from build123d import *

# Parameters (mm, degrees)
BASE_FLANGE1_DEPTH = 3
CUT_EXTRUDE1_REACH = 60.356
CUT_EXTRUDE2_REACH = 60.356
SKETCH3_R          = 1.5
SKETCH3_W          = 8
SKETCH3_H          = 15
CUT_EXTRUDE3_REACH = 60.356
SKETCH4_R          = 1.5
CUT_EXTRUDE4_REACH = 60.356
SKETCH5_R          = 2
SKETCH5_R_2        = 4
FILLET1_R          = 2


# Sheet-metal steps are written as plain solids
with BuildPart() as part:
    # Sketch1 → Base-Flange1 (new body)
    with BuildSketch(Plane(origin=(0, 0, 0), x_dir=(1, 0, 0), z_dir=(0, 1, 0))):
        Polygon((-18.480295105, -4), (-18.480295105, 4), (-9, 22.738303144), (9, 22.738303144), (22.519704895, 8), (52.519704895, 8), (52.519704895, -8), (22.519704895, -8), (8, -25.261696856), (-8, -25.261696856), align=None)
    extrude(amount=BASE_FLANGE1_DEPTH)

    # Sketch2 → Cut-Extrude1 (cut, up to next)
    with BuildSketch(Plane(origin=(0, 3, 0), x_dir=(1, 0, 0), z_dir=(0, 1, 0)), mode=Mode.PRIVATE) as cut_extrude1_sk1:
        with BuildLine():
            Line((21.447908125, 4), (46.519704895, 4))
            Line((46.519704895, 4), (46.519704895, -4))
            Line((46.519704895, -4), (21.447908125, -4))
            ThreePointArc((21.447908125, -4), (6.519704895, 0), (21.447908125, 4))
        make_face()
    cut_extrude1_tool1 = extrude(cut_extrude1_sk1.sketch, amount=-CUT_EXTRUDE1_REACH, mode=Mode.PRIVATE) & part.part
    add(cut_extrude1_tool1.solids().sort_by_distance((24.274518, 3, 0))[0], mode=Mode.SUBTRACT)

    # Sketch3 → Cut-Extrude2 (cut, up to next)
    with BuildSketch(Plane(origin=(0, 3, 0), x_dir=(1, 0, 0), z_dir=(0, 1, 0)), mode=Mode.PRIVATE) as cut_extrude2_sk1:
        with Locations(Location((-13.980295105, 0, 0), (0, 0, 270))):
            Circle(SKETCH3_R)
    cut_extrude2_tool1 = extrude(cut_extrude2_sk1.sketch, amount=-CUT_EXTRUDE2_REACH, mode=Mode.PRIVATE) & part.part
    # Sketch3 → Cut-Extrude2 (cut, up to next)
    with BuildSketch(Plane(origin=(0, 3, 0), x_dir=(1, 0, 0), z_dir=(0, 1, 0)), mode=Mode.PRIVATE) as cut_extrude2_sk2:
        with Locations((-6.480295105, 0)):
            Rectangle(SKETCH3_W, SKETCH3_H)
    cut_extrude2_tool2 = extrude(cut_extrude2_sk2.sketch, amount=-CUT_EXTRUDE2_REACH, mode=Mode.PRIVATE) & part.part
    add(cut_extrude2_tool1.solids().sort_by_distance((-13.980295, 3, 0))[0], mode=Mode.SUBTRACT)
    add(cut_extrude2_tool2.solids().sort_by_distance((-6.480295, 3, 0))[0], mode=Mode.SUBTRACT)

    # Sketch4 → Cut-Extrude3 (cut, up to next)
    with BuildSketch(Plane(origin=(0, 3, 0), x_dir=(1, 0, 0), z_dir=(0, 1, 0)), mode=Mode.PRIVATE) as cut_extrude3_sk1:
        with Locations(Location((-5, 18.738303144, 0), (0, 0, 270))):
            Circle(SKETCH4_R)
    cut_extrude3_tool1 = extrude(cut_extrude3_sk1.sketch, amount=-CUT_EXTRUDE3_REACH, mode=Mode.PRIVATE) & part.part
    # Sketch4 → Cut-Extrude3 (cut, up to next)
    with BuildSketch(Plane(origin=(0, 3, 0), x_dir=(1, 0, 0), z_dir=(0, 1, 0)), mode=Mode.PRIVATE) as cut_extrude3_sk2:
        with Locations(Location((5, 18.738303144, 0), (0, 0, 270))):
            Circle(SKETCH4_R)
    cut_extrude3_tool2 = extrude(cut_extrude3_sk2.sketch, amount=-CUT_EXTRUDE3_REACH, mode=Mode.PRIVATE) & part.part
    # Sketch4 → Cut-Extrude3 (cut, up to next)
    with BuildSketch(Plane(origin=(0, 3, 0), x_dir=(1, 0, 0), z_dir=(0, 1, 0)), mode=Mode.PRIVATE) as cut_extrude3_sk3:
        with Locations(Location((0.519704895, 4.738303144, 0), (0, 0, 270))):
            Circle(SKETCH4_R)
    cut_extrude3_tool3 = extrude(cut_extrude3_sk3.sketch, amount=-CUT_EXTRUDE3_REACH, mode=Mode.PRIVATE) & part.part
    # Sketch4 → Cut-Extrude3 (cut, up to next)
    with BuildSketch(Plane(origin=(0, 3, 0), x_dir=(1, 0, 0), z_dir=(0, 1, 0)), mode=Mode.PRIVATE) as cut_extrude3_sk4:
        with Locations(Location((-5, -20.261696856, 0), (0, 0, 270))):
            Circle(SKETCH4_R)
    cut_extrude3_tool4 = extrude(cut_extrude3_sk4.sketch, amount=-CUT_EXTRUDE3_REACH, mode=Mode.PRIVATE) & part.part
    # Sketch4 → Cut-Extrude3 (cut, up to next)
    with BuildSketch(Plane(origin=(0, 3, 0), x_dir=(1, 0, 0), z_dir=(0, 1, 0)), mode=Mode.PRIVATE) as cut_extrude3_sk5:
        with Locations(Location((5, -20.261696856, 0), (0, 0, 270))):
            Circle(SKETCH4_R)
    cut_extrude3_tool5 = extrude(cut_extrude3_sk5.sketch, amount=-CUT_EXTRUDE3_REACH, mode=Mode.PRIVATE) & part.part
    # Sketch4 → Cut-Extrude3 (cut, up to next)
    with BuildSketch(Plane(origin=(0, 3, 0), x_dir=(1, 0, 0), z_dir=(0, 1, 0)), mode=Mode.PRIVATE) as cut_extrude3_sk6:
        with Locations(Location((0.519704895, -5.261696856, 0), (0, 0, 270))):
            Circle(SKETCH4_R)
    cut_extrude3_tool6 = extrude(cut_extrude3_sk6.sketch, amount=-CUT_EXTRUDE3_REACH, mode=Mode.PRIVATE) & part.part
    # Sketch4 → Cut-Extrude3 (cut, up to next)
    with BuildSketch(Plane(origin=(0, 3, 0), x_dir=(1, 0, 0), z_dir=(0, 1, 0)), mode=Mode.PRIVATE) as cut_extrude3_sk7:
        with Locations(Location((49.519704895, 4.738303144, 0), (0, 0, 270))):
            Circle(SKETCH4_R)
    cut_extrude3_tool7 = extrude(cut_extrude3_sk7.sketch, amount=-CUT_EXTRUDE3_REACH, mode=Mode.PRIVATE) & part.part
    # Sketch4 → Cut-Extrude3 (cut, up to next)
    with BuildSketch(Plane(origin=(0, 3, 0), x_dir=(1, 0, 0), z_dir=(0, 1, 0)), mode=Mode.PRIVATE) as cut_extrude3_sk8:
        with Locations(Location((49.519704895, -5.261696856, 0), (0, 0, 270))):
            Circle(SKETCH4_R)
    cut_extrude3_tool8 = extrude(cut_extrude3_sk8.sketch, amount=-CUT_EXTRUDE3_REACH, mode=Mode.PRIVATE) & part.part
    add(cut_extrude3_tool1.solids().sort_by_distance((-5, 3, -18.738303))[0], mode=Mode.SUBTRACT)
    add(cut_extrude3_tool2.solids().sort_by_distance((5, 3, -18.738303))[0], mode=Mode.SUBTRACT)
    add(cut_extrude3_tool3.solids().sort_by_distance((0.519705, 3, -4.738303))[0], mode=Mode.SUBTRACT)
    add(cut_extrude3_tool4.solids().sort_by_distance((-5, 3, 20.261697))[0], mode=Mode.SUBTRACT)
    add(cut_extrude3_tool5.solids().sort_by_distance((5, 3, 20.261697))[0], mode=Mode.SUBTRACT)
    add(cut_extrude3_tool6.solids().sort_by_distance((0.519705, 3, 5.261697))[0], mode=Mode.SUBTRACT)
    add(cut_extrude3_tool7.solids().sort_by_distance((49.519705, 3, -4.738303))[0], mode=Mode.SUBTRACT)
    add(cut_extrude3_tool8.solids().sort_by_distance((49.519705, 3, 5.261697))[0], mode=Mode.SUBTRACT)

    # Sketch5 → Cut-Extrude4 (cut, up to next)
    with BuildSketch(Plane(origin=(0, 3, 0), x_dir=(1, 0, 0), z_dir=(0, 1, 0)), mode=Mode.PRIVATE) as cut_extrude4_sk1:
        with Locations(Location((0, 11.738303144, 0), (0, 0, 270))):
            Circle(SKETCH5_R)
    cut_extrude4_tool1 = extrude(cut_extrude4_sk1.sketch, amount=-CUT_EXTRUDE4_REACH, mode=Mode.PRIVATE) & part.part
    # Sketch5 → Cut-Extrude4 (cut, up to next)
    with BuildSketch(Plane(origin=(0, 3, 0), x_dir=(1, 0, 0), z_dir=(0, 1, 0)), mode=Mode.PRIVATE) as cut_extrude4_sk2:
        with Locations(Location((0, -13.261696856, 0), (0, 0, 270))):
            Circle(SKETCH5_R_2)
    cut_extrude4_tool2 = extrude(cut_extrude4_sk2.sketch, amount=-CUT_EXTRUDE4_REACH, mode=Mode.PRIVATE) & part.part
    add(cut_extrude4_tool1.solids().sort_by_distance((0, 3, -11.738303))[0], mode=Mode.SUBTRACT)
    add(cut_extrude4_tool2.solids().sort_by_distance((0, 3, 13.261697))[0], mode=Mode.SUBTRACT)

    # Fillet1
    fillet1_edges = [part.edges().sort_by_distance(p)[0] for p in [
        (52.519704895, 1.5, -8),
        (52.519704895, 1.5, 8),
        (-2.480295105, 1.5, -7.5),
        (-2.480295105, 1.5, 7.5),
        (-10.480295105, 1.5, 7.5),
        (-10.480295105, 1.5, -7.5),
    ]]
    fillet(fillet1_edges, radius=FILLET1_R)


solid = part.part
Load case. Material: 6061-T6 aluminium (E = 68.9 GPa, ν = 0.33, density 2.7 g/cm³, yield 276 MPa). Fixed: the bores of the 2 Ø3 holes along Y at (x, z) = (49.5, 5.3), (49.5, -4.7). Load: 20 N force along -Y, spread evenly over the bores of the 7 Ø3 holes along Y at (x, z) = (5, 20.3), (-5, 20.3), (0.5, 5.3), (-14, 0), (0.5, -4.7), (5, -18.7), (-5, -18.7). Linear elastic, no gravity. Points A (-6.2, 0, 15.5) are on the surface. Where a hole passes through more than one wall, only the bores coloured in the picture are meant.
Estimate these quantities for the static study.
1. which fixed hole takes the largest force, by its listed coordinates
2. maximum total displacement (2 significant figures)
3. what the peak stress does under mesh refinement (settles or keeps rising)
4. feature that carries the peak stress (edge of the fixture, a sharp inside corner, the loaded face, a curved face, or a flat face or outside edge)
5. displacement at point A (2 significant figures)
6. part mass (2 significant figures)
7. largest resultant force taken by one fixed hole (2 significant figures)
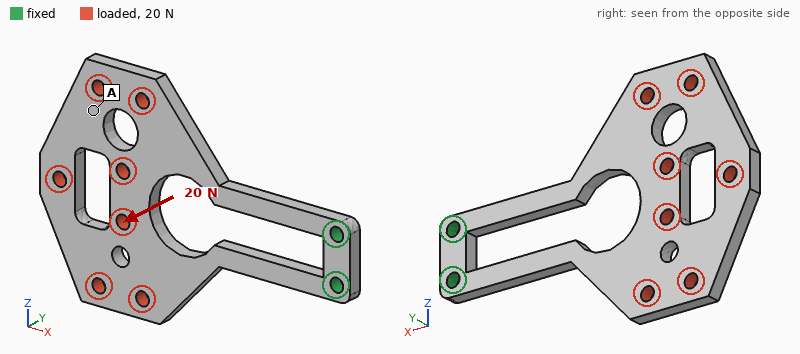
(49.5, 5.3)
1.00 mm
keeps rising
edge of the fixture
0.76 mm
11 g
11 N
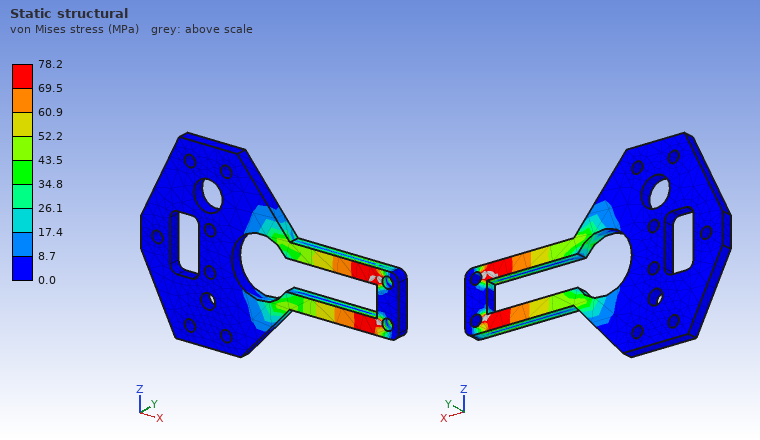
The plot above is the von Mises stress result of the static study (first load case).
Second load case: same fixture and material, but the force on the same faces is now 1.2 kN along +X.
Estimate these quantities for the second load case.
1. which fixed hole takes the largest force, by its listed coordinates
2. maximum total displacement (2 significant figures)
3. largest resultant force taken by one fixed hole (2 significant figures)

(49.5, 5.3)
86 µm
630 N
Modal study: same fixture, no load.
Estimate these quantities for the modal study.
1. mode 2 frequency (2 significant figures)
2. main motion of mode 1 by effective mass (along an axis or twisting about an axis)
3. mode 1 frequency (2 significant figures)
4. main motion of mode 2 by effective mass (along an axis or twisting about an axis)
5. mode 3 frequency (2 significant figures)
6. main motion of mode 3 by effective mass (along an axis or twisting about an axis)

760 Hz
along Y
300 Hz
twisting about X
820 Hz
along Z
